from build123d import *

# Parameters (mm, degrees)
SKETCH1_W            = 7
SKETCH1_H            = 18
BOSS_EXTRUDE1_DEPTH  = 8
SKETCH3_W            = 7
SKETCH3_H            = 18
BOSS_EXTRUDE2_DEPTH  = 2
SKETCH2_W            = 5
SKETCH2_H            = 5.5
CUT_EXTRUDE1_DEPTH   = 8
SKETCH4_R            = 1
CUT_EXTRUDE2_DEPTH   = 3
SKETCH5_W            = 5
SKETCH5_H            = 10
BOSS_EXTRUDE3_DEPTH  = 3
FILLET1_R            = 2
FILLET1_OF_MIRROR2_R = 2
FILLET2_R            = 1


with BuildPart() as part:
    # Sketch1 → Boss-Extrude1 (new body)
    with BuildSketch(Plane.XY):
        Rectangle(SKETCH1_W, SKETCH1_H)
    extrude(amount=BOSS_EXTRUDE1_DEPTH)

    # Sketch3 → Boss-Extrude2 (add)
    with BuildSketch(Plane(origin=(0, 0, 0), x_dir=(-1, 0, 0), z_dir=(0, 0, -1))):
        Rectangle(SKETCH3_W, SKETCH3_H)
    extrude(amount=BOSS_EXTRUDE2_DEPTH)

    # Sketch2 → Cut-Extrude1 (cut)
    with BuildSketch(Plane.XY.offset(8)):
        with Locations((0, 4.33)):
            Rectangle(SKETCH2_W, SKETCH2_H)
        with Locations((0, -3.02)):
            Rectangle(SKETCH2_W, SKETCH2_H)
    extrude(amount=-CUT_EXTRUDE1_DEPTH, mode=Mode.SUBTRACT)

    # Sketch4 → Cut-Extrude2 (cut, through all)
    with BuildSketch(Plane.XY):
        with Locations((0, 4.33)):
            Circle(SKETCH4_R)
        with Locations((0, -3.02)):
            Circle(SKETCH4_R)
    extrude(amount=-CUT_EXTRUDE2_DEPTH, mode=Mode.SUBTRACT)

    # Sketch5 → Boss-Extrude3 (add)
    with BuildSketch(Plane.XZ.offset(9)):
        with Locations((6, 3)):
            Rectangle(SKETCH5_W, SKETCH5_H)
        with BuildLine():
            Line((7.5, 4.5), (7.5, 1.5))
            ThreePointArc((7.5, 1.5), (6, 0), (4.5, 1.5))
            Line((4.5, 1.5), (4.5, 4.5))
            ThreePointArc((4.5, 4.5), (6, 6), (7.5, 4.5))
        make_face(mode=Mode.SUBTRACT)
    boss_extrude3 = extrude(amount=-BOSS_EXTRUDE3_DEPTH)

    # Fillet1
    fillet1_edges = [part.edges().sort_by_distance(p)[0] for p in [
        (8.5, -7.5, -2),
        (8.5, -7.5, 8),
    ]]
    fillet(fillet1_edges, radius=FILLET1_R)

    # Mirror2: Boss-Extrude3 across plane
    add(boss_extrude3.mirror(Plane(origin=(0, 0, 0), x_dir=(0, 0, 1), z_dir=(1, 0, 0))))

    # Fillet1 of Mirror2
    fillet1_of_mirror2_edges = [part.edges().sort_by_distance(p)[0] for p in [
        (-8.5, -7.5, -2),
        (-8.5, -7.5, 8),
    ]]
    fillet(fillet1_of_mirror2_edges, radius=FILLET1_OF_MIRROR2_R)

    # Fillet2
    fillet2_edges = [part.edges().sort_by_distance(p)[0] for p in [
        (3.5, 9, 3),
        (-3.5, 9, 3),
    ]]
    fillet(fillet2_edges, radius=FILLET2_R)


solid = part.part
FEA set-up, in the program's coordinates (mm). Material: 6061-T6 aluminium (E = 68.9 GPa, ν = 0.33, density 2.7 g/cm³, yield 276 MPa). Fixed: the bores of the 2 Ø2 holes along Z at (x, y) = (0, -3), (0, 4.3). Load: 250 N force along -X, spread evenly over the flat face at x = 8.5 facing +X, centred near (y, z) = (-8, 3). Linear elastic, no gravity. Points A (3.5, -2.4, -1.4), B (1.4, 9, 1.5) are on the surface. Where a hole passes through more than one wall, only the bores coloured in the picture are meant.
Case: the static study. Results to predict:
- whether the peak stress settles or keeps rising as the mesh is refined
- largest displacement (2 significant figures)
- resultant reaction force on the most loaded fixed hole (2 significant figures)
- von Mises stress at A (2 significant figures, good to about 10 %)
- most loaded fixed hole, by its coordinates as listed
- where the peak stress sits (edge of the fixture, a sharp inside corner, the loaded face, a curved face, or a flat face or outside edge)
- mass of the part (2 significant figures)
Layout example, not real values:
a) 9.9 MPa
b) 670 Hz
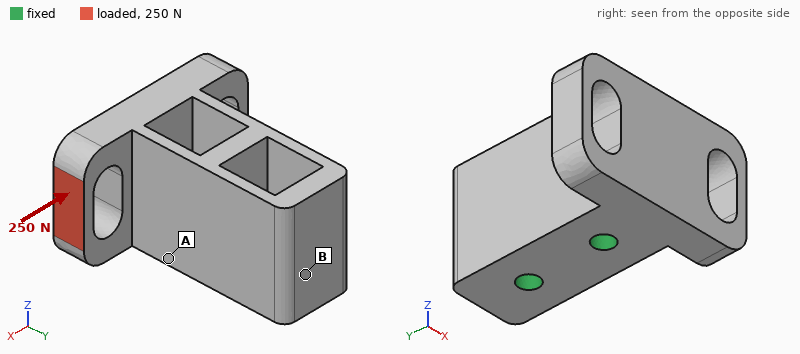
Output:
a) keeps rising
b) 35 µm
c) 330 N
d) 38 MPa
e) (0, -3)
f) edge of the fixture
g) 2.7 g
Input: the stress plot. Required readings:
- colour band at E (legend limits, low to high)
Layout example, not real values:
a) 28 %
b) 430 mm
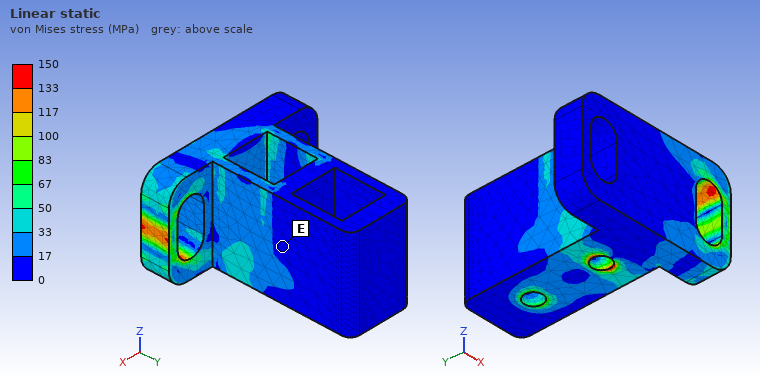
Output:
a) 0 to 17 MPa
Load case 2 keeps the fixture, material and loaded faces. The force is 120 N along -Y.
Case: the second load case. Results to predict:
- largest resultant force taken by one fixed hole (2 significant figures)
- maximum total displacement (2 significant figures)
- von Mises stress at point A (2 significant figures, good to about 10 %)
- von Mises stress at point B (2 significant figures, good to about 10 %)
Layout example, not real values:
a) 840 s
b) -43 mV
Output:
a) 130 N
b) 30 µm
c) 18 MPa
d) 6.1 MPa
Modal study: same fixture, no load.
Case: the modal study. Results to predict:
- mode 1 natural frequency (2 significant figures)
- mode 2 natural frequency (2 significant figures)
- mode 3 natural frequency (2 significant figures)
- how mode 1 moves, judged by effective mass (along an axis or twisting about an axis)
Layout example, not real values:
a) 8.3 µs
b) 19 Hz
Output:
a) 13 kHz
b) 22 kHz
c) 25 kHz
d) along X
